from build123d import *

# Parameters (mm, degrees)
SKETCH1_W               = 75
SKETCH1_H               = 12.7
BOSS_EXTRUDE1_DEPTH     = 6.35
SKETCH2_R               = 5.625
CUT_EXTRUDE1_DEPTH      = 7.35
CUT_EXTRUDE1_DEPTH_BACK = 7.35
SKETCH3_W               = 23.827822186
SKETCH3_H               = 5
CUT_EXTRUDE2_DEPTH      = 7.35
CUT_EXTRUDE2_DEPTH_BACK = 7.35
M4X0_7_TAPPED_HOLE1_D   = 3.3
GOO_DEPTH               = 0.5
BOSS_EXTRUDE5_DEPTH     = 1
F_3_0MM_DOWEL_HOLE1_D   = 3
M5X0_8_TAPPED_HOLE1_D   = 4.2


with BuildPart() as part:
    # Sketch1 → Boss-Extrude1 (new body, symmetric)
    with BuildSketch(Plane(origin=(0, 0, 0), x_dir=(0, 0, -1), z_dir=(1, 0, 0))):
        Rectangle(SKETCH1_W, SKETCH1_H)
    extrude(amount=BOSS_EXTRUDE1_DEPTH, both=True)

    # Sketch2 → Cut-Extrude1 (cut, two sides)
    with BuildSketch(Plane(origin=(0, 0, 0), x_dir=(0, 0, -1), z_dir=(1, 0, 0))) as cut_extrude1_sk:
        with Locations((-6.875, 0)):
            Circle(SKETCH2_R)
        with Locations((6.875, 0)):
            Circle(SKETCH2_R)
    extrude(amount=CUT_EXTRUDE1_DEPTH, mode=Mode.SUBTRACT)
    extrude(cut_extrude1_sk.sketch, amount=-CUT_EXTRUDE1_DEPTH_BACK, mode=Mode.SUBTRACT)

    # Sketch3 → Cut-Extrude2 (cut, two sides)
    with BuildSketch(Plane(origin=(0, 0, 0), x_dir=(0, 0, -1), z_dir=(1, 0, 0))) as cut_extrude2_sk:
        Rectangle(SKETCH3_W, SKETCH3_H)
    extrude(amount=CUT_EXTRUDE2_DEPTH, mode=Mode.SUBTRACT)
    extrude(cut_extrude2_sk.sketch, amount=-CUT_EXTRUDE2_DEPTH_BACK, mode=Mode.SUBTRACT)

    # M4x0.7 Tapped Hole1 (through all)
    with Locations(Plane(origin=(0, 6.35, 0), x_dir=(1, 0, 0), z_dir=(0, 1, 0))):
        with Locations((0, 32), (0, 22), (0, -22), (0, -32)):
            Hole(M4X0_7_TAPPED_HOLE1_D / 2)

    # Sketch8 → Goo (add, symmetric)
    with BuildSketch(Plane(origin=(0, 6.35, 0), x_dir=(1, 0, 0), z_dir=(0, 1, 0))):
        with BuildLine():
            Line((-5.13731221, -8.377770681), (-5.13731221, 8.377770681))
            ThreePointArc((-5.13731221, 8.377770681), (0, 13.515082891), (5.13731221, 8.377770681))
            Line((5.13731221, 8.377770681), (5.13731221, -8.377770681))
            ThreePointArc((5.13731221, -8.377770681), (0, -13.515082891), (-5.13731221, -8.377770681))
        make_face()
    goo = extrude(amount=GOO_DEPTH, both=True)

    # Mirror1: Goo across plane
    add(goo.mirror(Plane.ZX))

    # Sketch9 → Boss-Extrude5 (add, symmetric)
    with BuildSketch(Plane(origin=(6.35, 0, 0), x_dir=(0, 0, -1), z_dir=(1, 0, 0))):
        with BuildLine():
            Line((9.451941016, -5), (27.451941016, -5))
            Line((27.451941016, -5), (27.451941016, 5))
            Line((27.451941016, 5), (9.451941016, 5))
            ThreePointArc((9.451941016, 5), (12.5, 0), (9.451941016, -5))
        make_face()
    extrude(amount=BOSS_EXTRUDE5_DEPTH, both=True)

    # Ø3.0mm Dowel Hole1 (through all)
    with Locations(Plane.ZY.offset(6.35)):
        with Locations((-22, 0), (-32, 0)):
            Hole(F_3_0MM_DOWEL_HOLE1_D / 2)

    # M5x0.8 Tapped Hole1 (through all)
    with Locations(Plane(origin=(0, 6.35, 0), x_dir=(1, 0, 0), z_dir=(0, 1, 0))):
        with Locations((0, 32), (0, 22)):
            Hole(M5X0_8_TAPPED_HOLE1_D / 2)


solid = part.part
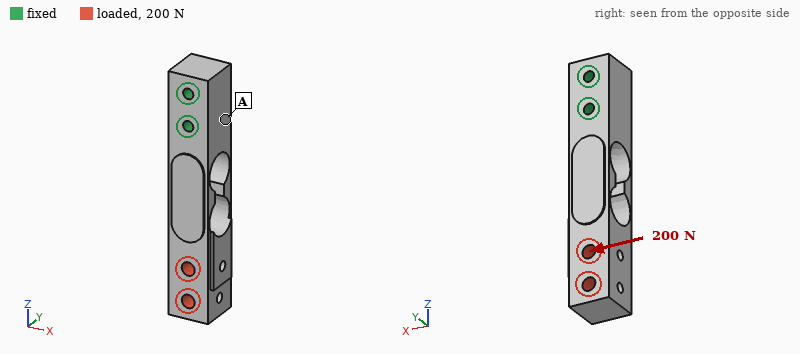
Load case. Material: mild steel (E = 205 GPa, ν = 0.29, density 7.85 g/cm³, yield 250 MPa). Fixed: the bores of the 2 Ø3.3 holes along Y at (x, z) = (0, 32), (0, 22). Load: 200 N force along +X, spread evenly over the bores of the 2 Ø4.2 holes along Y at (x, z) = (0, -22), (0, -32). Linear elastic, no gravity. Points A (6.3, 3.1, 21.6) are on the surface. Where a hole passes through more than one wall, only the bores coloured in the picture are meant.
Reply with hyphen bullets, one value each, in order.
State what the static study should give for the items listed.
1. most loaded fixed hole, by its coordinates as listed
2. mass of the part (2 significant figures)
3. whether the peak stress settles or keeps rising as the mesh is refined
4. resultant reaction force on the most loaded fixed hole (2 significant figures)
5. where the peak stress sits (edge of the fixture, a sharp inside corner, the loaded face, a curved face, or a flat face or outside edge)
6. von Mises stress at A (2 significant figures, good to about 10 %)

- (0, 22)
- 71 g
- keeps rising
- 750 N
- a sharp inside corner
- 23 MPa
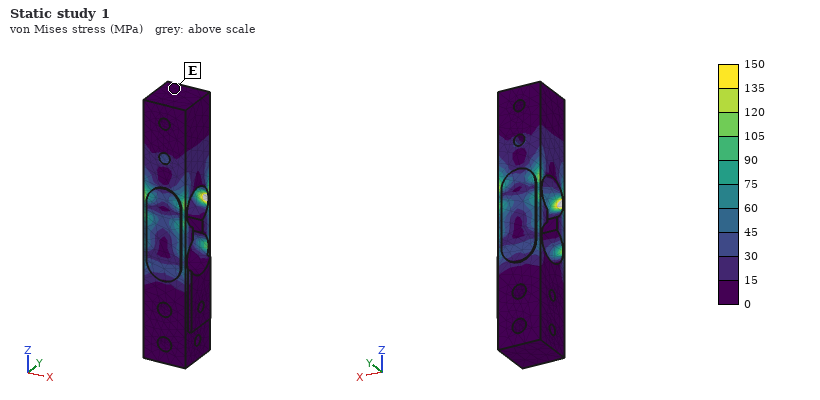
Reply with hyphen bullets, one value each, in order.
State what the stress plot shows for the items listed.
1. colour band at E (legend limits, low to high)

- 0 to 15 MPa
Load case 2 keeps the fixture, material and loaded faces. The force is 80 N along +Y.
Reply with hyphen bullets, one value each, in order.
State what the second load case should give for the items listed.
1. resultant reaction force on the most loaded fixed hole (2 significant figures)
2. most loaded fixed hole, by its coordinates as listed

- 130 N
- (0, 22)
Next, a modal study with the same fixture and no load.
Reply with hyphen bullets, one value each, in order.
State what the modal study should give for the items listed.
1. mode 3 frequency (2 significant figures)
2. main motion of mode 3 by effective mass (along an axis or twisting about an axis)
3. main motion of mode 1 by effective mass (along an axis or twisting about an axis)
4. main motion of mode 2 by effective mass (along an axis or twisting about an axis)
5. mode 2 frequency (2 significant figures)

- 5800 Hz
- twisting about Z
- along Y
- along X
- 1700 Hz
